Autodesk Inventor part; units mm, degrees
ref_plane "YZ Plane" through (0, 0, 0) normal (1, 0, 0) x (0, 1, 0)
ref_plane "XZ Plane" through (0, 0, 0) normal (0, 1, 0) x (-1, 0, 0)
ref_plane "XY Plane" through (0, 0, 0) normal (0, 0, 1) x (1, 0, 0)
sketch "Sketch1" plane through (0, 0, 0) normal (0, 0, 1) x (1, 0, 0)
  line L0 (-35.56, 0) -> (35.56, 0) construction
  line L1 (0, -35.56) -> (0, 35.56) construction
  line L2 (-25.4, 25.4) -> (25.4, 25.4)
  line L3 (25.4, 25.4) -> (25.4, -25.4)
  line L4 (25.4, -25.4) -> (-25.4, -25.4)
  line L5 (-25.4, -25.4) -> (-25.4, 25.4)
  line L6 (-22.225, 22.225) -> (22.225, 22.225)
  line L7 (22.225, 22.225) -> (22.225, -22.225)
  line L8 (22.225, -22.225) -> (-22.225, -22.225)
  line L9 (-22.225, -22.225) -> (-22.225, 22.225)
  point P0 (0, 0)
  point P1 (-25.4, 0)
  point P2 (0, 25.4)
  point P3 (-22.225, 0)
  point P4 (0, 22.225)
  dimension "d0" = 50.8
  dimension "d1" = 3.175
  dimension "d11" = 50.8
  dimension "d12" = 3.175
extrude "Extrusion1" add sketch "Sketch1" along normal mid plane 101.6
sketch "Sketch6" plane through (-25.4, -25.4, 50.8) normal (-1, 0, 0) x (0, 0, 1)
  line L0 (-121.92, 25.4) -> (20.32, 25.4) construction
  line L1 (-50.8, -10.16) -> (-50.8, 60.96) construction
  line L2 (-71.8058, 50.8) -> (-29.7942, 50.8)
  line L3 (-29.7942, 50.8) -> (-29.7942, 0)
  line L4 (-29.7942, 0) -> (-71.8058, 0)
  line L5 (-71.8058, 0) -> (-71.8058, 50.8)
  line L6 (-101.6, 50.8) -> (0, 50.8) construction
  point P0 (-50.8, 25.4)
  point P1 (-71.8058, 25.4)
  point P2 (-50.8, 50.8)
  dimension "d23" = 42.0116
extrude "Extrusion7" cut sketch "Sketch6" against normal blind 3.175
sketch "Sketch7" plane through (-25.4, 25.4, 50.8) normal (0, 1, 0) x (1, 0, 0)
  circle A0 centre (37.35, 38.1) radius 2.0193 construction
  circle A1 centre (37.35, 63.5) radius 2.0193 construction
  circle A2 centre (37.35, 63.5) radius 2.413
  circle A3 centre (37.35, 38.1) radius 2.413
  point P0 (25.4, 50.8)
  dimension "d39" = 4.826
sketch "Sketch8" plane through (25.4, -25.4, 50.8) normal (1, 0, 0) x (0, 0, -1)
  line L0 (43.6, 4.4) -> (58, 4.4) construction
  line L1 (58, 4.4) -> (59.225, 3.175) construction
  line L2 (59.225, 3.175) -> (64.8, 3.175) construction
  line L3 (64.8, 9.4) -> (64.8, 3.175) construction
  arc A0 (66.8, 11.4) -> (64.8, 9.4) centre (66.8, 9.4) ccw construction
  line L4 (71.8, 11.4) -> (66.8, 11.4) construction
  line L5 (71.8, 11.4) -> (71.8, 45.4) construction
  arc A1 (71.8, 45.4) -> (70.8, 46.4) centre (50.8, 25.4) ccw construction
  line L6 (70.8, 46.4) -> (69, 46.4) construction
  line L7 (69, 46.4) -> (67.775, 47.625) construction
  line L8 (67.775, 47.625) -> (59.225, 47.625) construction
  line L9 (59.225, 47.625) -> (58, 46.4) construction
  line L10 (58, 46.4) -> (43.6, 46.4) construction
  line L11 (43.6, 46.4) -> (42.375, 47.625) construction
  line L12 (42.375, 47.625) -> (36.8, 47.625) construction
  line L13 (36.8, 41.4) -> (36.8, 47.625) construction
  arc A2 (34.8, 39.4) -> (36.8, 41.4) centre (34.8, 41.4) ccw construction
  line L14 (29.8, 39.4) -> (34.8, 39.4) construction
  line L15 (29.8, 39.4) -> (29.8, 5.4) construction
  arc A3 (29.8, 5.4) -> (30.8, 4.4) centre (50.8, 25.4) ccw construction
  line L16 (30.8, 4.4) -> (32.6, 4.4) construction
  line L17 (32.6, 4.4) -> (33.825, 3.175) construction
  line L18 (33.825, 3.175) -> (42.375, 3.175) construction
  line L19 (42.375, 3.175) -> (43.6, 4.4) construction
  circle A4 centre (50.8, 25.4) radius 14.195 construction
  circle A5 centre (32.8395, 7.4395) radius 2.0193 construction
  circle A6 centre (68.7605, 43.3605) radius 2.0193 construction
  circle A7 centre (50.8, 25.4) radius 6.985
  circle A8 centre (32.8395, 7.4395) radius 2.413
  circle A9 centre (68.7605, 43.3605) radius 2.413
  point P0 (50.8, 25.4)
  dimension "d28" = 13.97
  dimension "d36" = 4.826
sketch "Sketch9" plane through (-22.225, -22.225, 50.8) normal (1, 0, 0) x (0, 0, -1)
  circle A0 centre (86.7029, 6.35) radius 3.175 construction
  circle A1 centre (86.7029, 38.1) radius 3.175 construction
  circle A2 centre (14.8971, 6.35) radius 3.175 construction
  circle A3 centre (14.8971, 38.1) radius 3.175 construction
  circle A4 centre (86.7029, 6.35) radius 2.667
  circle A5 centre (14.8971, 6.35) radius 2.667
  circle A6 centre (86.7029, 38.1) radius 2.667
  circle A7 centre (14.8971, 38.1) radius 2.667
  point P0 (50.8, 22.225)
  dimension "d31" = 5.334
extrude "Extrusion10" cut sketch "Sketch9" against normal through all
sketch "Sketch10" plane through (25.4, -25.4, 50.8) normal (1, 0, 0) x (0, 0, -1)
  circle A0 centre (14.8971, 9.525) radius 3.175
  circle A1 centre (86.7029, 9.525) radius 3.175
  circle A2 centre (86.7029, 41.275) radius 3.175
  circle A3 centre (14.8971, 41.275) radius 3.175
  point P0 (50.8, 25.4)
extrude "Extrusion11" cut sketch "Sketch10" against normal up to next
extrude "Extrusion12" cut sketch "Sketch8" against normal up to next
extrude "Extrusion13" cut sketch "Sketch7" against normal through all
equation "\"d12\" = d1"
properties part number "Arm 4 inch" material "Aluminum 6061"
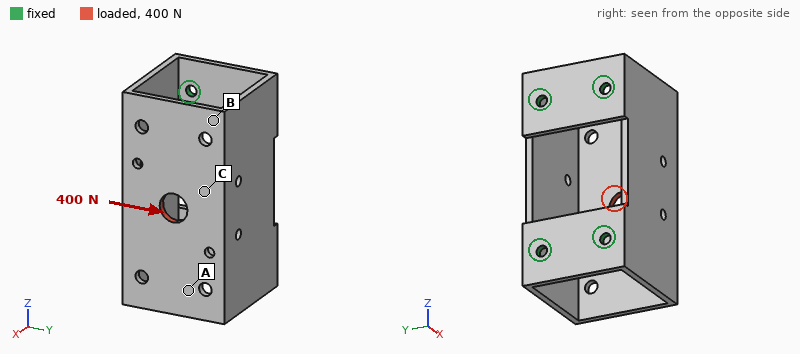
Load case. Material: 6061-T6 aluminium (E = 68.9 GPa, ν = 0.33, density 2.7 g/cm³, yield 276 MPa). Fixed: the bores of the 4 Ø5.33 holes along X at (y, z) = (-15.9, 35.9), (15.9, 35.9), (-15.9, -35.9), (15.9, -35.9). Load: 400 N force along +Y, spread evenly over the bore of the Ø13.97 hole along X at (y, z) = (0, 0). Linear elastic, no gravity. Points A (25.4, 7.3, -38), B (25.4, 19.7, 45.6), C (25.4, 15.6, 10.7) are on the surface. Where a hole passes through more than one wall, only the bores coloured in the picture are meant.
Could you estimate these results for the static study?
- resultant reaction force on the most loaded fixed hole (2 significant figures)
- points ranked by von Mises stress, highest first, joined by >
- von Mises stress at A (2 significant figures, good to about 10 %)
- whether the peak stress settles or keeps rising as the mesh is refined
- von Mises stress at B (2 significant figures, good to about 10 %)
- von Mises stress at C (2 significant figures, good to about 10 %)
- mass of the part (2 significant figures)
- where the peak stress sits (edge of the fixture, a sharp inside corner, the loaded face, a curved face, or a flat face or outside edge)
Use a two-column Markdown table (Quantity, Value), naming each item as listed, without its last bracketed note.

| Quantity | Value |
|---|---|
| resultant reaction force on the most loaded fixed hole | 180 N |
| points ranked by von Mises stress, highest first, joined by > | B > C > A |
| von Mises stress at A | 6.9 MPa |
| whether the peak stress settles or keeps rising as the mesh is refined | keeps rising |
| von Mises stress at B | 26 MPa |
| von Mises stress at C | 18 MPa |
| mass of the part | 140 g |
| where the peak stress sits | edge of the fixture |
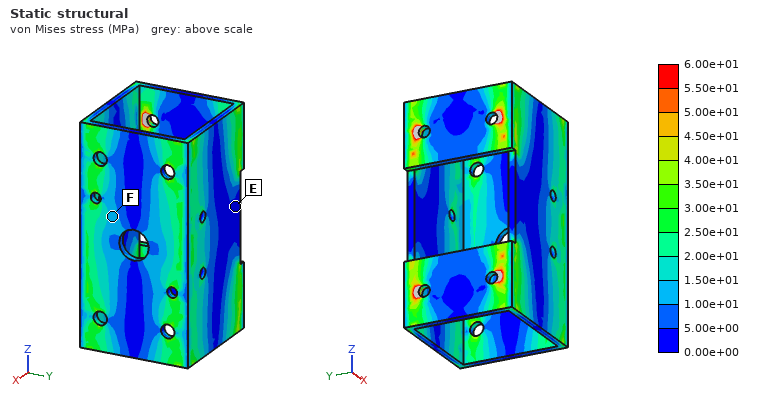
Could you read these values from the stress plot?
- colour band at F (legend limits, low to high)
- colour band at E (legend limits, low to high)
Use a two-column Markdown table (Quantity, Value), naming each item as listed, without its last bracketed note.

| Quantity | Value |
|---|---|
| colour band at F | 1.00e+01 to 1.50e+01 MPa |
| colour band at E | 0.00e+00 to 5.00e+00 MPa |
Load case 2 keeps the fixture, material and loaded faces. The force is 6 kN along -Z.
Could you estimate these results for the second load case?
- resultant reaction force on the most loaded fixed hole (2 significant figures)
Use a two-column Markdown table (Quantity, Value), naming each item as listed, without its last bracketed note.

| Quantity | Value |
|---|---|
| resultant reaction force on the most loaded fixed hole | 2.5 kN |
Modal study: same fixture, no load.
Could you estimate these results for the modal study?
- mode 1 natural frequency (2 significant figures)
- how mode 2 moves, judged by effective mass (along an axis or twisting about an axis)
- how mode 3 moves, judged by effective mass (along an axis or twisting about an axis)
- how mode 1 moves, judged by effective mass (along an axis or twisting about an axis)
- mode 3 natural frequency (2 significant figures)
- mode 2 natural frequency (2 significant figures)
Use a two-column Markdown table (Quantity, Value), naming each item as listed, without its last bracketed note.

| Quantity | Value |
|---|---|
| mode 1 natural frequency | 770 Hz |
| how mode 2 moves, judged by effective mass | along X |
| how mode 3 moves, judged by effective mass | along Z |
| how mode 1 moves, judged by effective mass | along Y |
| mode 3 natural frequency | 3400 Hz |
| mode 2 natural frequency | 3200 Hz |
